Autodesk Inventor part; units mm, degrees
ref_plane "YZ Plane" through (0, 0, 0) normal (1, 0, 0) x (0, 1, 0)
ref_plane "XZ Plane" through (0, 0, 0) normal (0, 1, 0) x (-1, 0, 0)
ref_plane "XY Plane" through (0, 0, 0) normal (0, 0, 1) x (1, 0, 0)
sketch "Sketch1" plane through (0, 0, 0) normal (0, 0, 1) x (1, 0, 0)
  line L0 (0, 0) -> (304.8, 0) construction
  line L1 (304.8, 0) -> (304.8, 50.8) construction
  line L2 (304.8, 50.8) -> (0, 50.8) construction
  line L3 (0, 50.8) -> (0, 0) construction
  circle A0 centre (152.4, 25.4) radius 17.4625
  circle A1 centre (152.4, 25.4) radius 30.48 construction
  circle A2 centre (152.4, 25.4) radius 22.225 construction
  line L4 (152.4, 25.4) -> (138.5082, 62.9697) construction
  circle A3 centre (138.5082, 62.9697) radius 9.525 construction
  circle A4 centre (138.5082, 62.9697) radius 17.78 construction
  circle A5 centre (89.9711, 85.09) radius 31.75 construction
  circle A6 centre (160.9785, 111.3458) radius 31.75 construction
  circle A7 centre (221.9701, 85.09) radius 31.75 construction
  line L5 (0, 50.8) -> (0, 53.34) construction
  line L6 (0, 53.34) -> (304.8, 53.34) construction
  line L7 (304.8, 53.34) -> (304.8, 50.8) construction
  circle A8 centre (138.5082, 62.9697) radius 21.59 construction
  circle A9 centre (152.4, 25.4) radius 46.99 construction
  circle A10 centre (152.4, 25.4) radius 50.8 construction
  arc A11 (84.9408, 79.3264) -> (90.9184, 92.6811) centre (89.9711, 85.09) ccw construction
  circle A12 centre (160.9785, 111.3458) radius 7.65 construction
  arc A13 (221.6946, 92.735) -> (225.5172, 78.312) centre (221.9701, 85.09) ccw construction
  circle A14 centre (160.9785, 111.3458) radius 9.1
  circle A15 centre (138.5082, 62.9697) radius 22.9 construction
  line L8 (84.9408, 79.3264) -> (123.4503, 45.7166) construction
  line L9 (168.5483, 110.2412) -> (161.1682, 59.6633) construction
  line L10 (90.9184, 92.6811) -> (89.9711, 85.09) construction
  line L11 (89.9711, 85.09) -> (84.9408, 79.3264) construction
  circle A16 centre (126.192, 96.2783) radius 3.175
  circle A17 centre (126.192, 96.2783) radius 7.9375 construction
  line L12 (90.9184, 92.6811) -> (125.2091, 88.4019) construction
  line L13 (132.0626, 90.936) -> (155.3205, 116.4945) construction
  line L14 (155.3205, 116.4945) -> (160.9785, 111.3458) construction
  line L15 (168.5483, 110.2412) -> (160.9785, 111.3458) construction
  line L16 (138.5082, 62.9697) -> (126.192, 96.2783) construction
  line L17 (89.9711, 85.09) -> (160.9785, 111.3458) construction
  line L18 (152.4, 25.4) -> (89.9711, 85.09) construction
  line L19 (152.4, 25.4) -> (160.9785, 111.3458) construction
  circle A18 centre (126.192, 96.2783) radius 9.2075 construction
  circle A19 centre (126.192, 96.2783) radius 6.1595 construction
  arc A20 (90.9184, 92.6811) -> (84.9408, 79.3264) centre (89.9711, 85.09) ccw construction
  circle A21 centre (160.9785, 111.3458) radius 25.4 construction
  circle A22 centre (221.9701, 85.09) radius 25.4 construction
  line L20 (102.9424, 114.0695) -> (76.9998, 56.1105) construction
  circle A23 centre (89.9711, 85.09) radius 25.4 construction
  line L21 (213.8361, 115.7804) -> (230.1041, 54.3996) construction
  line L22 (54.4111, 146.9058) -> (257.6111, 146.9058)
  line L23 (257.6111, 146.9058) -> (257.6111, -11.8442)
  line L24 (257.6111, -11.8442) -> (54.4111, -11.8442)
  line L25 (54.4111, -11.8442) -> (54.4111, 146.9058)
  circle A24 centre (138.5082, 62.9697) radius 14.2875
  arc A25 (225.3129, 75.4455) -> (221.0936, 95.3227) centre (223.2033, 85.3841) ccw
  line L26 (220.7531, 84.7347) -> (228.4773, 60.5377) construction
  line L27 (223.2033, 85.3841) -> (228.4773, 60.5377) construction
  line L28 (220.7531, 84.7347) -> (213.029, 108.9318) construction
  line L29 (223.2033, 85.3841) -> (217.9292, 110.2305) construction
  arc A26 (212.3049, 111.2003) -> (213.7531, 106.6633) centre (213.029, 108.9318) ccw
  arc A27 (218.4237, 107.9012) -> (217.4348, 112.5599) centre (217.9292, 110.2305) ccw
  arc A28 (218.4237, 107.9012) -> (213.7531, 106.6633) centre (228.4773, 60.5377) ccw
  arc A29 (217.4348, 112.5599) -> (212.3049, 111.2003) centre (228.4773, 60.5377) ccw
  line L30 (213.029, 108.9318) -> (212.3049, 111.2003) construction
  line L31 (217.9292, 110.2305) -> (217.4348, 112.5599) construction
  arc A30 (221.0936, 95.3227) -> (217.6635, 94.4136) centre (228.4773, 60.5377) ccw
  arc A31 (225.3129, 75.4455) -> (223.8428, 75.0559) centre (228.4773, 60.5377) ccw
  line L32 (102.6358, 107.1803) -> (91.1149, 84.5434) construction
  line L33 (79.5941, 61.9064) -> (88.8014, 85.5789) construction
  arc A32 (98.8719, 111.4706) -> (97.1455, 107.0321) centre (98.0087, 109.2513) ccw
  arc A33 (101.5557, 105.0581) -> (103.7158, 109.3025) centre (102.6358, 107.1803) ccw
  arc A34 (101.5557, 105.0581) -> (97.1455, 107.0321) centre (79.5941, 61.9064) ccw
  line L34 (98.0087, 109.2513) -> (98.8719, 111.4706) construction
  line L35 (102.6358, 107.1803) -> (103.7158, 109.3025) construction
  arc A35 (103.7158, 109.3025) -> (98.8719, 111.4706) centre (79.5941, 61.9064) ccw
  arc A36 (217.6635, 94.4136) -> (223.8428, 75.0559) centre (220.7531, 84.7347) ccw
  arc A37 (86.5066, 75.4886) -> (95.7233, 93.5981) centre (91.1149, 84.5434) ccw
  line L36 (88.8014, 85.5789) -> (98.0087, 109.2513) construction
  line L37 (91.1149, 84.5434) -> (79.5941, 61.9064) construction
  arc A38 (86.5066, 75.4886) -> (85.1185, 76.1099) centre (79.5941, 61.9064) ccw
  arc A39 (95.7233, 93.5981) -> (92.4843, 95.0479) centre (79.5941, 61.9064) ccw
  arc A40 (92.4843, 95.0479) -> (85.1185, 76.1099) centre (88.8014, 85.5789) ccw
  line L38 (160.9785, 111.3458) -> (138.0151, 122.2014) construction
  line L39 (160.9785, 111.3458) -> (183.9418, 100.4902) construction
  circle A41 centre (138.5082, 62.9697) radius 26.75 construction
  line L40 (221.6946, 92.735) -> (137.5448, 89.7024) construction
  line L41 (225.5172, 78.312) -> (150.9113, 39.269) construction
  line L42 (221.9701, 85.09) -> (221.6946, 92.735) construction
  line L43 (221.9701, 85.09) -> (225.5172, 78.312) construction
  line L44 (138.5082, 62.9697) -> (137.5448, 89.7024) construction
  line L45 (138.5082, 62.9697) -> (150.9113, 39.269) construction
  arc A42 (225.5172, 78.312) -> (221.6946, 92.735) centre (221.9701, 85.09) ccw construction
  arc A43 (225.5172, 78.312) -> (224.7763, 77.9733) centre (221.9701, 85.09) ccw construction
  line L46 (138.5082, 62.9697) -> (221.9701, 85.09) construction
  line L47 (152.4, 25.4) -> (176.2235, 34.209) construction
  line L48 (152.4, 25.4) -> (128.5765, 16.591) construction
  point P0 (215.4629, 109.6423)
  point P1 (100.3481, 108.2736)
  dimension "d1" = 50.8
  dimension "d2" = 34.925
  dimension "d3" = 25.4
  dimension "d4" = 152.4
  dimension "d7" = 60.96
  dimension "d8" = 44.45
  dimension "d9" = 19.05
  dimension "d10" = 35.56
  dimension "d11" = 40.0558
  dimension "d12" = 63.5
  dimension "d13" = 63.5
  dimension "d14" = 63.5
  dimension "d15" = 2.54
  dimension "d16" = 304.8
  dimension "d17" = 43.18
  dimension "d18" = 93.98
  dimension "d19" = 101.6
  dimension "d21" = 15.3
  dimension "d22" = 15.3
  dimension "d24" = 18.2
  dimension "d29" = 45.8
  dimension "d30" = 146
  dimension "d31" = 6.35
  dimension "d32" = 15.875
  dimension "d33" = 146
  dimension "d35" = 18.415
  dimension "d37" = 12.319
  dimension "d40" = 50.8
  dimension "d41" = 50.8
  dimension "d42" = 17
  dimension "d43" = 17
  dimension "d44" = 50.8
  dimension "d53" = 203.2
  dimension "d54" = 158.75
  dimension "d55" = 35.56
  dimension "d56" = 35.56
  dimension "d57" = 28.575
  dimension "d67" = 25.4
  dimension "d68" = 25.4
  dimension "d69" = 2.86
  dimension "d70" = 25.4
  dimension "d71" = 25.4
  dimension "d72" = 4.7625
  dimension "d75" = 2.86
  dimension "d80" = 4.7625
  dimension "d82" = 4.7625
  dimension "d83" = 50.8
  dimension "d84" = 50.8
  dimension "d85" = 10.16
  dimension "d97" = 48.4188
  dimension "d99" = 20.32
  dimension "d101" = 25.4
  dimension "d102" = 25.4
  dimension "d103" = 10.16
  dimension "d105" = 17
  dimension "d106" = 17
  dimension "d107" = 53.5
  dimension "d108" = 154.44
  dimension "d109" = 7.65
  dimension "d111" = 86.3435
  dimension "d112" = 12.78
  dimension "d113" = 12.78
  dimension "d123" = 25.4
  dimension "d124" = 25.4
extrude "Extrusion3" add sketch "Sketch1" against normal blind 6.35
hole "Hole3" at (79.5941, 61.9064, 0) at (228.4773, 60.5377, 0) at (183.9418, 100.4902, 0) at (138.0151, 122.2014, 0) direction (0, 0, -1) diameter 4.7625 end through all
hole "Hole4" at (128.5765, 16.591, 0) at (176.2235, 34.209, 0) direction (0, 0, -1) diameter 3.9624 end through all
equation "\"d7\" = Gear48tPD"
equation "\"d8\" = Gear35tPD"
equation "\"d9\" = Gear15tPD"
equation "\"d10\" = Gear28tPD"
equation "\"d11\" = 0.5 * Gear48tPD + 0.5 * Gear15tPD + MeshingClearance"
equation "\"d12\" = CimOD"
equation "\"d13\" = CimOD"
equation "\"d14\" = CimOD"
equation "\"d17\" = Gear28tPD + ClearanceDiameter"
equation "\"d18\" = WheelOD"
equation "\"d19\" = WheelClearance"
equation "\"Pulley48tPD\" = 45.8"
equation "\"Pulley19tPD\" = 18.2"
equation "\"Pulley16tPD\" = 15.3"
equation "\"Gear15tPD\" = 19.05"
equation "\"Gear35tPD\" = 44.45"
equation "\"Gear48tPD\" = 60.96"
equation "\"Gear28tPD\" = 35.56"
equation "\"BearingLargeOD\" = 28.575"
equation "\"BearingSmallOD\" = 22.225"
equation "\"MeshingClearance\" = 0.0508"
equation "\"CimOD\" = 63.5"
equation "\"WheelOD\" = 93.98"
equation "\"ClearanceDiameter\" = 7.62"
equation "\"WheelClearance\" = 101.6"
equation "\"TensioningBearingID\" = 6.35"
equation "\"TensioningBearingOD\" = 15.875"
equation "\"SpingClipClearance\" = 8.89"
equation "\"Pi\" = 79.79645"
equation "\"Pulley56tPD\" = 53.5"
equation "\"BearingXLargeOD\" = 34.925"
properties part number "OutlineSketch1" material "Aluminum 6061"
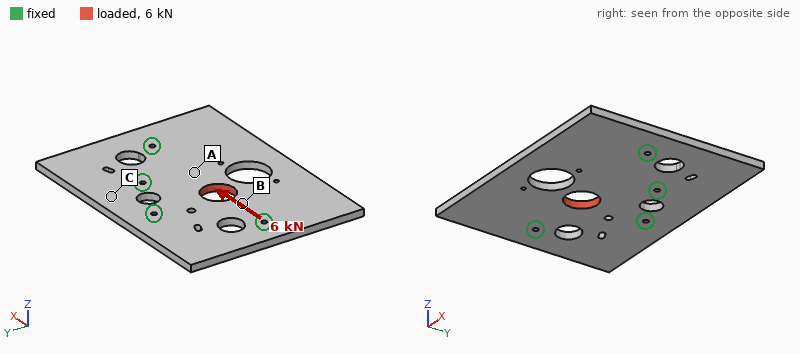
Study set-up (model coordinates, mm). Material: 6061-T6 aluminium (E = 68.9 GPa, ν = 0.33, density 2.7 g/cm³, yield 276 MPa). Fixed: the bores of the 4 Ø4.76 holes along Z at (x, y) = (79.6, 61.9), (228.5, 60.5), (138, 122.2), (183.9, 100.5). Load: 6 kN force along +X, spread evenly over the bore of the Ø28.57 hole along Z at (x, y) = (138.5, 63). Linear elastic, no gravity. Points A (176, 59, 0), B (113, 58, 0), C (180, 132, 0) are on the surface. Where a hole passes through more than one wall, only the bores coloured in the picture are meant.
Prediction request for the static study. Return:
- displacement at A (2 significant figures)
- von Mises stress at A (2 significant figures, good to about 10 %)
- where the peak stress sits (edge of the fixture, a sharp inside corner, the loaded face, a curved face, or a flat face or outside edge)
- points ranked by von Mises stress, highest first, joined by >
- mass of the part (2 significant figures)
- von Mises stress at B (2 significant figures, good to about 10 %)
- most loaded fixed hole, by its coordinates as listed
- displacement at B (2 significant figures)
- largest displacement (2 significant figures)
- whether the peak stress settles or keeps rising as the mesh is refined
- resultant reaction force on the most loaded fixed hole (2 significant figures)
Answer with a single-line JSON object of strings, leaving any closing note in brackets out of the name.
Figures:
{"displacement at A": "6.2 µm", "von Mises stress at A": "7.6 MPa", "where the peak stress sits": "edge of the fixture", "points ranked by von Mises stress, highest first, joined by >": "B > A > C", "mass of the part": "500 g", "von Mises stress at B": "12 MPa", "most loaded fixed hole, by its coordinates as listed": "(79.6, 61.9)", "displacement at B": "7.0 µm", "largest displacement": "11 µm", "whether the peak stress settles or keeps rising as the mesh is refined": "keeps rising", "resultant reaction force on the most loaded fixed hole": "2.5 kN"}
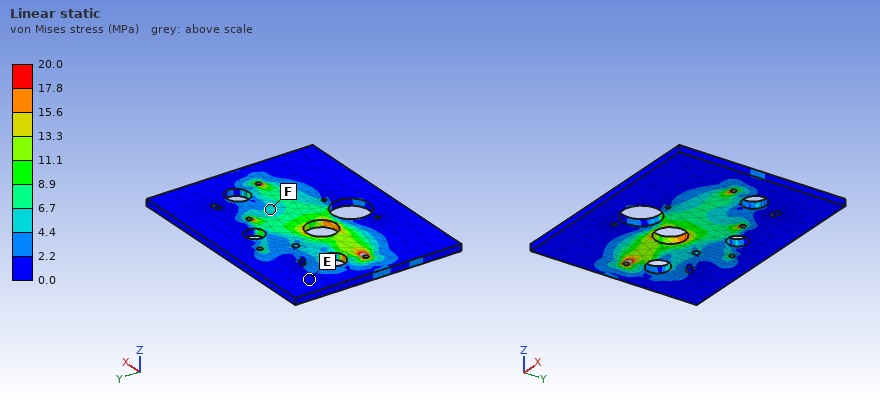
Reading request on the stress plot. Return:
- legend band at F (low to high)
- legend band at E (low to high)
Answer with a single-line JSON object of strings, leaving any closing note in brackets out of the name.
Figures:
{"legend band at F": "4.4 to 6.7 MPa", "legend band at E": "0.0 to 2.2 MPa"}
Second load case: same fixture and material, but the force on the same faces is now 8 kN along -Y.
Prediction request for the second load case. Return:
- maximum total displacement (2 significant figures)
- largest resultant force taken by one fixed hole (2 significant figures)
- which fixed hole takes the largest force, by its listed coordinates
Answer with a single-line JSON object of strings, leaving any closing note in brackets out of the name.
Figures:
{"maximum total displacement": "23 µm", "largest resultant force taken by one fixed hole": "3.0 kN", "which fixed hole takes the largest force, by its listed coordinates": "(138, 122.2)"}
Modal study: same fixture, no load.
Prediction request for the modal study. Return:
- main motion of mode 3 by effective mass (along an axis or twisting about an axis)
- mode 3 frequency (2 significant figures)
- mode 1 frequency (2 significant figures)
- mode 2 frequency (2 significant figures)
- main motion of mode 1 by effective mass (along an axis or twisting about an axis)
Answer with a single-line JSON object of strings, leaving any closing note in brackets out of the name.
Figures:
{"main motion of mode 3 by effective mass": "along Z", "mode 3 frequency": "1200 Hz", "mode 1 frequency": "680 Hz", "mode 2 frequency": "1100 Hz", "main motion of mode 1 by effective mass": "along Z"}
